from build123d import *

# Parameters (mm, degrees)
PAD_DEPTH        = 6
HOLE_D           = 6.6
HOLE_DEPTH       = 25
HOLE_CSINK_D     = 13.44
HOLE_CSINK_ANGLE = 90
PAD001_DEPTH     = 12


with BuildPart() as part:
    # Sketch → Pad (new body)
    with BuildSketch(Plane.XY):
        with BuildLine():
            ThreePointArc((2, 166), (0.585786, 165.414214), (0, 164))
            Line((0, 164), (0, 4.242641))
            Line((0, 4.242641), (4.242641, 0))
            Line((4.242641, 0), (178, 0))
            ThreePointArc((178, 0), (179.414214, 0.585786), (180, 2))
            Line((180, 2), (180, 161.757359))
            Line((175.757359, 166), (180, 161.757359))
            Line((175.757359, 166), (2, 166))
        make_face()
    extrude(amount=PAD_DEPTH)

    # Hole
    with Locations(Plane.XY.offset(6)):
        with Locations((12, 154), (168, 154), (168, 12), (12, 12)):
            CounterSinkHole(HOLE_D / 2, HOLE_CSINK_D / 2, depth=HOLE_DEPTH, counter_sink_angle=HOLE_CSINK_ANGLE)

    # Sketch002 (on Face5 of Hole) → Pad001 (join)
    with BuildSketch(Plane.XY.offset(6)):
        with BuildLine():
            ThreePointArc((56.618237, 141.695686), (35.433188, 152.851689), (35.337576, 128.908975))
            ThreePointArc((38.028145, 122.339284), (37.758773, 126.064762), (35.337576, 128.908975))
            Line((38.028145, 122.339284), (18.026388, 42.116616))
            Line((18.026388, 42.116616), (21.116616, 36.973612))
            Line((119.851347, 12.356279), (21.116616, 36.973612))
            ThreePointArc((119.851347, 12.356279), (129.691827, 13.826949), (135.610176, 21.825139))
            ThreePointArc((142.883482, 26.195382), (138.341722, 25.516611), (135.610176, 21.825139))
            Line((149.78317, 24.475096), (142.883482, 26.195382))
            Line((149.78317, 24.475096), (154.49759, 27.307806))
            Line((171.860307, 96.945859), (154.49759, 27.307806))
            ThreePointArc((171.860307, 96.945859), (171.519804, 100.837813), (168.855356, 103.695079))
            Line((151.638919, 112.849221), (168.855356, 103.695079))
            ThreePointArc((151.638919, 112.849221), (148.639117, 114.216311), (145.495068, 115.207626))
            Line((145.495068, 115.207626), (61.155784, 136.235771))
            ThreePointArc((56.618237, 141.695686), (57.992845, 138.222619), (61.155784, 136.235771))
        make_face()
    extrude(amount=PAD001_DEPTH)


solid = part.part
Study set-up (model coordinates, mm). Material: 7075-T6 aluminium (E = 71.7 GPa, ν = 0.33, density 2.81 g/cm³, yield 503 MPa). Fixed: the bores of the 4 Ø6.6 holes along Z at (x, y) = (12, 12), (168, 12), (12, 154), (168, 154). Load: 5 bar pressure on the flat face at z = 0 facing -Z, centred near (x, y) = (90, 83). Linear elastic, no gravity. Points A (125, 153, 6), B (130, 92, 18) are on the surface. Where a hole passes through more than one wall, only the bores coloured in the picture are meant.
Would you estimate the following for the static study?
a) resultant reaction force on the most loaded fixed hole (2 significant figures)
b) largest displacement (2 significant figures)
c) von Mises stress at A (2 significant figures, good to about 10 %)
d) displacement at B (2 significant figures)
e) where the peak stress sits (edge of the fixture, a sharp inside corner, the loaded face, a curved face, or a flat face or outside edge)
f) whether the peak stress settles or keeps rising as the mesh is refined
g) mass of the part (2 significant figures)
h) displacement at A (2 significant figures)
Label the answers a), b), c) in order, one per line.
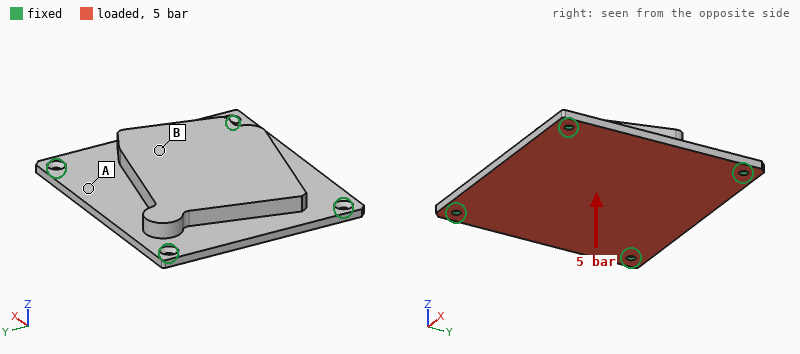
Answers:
a) 9.4 kN
b) 0.44 mm
c) 67 MPa
d) 0.36 mm
e) edge of the fixture
f) keeps rising
g) 990 g
h) 0.34 mm
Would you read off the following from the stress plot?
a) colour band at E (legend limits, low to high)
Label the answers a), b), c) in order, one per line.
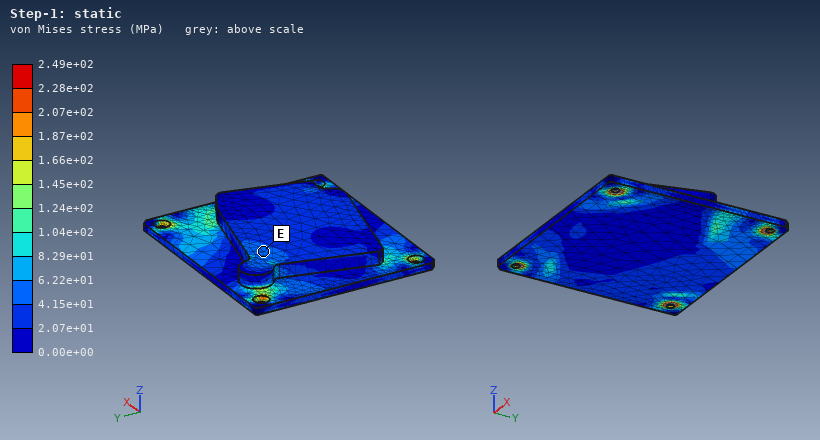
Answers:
a) 4.15e+01 to 6.22e+01 MPa
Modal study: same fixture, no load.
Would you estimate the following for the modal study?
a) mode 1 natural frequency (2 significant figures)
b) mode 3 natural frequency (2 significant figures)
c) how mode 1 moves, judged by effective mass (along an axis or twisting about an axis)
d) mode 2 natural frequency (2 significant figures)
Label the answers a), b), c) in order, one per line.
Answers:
a) 1100 Hz
b) 2000 Hz
c) along Z
d) 1600 Hz
